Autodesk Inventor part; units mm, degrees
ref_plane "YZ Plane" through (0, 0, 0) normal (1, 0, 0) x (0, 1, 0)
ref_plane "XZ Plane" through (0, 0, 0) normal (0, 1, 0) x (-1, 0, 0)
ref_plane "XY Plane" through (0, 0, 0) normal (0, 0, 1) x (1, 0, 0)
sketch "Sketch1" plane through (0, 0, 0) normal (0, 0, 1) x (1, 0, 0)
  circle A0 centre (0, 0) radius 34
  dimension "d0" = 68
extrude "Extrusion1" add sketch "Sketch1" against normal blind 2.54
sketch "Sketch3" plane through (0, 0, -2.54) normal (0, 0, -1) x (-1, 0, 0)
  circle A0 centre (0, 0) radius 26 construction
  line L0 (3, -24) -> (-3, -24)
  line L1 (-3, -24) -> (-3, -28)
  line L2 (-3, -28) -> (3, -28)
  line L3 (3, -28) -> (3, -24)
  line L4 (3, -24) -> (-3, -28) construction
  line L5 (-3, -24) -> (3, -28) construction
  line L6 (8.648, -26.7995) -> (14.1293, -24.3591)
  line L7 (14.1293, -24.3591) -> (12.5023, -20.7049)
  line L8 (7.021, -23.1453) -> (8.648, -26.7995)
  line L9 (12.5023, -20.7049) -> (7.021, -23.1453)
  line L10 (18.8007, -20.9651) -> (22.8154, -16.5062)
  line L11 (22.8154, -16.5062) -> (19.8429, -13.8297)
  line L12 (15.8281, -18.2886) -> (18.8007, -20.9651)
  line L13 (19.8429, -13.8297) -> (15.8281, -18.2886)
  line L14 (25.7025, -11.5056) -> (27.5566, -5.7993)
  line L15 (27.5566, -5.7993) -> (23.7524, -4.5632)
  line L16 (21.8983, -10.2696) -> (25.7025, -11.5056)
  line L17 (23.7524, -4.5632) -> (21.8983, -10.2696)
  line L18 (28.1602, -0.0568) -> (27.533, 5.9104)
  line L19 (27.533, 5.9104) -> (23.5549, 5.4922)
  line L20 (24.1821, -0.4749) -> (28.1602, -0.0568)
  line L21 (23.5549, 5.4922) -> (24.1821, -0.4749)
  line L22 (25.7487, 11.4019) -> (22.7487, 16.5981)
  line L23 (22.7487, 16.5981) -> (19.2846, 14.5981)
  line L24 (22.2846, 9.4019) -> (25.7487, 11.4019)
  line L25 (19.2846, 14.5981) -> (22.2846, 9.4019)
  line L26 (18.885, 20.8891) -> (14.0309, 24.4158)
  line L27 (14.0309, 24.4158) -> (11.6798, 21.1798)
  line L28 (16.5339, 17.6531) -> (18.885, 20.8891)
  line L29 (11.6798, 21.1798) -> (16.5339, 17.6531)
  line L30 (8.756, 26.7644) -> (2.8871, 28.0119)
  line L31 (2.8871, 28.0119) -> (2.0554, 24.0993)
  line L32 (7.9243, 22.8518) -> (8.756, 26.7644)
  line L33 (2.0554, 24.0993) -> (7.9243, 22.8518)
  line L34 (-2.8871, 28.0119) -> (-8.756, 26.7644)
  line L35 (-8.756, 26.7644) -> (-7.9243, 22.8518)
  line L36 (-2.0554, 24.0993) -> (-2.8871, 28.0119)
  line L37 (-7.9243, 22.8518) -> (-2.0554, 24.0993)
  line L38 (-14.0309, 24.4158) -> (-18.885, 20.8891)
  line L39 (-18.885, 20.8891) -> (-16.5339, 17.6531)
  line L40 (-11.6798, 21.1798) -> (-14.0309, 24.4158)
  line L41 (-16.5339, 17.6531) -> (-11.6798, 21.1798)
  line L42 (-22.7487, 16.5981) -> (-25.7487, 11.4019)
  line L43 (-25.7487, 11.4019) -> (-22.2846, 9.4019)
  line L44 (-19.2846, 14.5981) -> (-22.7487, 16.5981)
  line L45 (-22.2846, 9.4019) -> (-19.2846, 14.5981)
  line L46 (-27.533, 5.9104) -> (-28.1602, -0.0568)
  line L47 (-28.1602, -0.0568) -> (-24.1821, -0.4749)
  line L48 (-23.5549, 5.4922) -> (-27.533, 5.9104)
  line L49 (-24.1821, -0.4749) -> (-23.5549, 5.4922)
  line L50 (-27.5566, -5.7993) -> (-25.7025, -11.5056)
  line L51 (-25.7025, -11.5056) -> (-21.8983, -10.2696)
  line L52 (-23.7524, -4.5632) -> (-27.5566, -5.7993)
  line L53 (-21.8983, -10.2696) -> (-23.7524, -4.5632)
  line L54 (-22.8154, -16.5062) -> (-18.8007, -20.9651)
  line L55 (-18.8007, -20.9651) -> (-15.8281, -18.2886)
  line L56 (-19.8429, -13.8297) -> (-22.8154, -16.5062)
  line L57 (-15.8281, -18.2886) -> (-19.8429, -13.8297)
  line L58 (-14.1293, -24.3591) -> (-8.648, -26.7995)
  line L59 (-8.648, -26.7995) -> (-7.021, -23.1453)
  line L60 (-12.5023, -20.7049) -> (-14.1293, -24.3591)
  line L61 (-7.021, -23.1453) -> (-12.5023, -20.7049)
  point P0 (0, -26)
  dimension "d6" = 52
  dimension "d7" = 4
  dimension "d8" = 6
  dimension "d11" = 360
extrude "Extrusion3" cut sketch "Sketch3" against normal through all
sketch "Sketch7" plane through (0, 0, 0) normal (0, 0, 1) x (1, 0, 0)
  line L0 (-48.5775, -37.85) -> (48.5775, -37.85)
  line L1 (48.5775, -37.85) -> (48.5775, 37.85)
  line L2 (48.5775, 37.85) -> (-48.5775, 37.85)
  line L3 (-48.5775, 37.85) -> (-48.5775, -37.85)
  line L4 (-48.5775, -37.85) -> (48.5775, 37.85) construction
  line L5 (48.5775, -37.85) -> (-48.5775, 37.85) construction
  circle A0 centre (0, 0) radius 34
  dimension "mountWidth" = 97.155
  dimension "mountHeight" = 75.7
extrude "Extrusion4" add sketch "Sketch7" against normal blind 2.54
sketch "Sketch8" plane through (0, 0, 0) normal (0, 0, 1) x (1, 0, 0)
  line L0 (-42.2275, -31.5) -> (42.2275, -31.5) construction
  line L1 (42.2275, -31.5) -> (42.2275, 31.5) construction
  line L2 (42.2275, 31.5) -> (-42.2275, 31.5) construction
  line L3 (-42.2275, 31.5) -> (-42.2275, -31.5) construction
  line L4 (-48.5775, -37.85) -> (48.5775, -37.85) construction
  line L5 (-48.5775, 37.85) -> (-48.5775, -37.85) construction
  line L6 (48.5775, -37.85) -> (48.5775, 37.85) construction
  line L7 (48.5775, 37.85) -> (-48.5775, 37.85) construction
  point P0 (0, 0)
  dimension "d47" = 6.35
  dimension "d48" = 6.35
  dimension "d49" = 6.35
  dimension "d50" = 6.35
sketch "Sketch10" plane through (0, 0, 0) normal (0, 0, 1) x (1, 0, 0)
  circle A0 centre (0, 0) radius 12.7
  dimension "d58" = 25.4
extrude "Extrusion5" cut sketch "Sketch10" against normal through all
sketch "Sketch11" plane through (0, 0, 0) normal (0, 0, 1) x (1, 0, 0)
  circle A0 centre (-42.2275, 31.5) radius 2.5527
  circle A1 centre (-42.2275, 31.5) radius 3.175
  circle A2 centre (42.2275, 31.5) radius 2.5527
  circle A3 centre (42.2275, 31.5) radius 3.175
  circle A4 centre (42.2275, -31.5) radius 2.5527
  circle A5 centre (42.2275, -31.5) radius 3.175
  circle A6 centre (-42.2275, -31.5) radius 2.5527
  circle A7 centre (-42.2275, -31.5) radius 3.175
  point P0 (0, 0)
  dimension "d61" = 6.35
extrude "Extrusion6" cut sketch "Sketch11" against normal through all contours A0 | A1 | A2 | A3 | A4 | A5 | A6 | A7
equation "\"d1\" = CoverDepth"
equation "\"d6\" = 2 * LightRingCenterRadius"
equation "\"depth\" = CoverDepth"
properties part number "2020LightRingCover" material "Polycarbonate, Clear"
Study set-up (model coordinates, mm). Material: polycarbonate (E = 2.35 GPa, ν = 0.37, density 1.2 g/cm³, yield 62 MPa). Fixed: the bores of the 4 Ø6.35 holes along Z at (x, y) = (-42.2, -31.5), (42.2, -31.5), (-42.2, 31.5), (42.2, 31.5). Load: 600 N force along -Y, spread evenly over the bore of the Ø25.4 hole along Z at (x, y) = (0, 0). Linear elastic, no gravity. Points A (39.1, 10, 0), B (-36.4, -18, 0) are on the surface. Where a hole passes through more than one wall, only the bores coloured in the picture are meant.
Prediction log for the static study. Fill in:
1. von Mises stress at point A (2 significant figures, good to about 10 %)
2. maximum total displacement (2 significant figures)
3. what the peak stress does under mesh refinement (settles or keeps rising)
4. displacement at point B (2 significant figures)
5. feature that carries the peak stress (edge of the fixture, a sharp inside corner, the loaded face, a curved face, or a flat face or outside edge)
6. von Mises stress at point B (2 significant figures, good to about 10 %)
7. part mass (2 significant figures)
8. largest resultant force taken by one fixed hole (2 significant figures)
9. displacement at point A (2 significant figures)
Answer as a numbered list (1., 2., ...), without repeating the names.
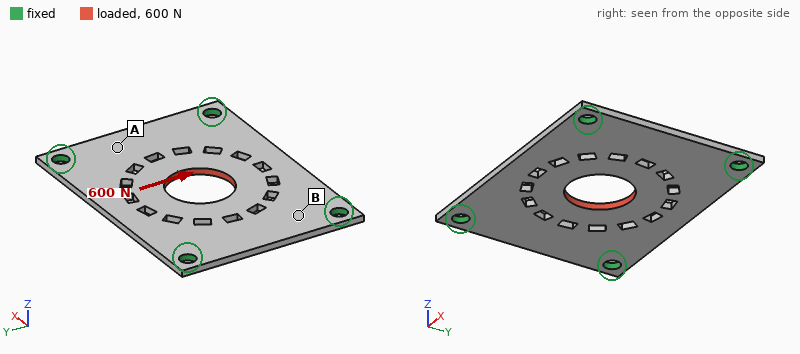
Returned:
1. 2.0 MPa
2. 0.12 mm
3. keeps rising
4. 0.023 mm
5. a sharp inside corner
6. 3.0 MPa
7. 19 g
8. 180 N
9. 0.023 mm
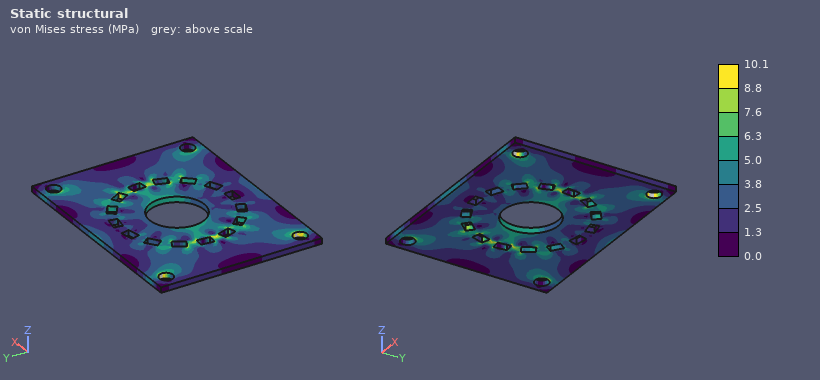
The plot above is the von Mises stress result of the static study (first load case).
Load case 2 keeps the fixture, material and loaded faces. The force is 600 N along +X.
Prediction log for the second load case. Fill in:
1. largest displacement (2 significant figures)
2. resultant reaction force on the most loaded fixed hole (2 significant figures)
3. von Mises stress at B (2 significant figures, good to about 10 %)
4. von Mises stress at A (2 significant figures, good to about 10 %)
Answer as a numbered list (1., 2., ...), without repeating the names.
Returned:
1. 76 µm
2. 160 N
3. 2.6 MPa
4. 1.3 MPa
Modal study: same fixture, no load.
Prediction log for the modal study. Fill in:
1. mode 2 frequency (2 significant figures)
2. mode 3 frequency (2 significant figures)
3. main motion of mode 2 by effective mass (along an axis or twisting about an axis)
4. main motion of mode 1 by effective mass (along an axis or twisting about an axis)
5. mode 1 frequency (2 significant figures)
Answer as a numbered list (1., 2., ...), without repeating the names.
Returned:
1. 660 Hz
2. 910 Hz
3. twisting about X
4. along Z
5. 470 Hz
